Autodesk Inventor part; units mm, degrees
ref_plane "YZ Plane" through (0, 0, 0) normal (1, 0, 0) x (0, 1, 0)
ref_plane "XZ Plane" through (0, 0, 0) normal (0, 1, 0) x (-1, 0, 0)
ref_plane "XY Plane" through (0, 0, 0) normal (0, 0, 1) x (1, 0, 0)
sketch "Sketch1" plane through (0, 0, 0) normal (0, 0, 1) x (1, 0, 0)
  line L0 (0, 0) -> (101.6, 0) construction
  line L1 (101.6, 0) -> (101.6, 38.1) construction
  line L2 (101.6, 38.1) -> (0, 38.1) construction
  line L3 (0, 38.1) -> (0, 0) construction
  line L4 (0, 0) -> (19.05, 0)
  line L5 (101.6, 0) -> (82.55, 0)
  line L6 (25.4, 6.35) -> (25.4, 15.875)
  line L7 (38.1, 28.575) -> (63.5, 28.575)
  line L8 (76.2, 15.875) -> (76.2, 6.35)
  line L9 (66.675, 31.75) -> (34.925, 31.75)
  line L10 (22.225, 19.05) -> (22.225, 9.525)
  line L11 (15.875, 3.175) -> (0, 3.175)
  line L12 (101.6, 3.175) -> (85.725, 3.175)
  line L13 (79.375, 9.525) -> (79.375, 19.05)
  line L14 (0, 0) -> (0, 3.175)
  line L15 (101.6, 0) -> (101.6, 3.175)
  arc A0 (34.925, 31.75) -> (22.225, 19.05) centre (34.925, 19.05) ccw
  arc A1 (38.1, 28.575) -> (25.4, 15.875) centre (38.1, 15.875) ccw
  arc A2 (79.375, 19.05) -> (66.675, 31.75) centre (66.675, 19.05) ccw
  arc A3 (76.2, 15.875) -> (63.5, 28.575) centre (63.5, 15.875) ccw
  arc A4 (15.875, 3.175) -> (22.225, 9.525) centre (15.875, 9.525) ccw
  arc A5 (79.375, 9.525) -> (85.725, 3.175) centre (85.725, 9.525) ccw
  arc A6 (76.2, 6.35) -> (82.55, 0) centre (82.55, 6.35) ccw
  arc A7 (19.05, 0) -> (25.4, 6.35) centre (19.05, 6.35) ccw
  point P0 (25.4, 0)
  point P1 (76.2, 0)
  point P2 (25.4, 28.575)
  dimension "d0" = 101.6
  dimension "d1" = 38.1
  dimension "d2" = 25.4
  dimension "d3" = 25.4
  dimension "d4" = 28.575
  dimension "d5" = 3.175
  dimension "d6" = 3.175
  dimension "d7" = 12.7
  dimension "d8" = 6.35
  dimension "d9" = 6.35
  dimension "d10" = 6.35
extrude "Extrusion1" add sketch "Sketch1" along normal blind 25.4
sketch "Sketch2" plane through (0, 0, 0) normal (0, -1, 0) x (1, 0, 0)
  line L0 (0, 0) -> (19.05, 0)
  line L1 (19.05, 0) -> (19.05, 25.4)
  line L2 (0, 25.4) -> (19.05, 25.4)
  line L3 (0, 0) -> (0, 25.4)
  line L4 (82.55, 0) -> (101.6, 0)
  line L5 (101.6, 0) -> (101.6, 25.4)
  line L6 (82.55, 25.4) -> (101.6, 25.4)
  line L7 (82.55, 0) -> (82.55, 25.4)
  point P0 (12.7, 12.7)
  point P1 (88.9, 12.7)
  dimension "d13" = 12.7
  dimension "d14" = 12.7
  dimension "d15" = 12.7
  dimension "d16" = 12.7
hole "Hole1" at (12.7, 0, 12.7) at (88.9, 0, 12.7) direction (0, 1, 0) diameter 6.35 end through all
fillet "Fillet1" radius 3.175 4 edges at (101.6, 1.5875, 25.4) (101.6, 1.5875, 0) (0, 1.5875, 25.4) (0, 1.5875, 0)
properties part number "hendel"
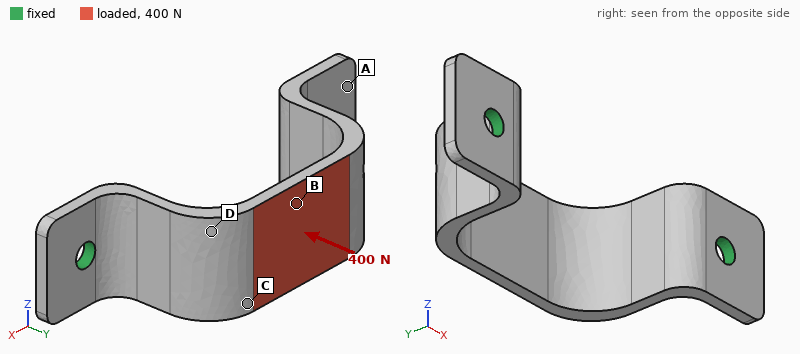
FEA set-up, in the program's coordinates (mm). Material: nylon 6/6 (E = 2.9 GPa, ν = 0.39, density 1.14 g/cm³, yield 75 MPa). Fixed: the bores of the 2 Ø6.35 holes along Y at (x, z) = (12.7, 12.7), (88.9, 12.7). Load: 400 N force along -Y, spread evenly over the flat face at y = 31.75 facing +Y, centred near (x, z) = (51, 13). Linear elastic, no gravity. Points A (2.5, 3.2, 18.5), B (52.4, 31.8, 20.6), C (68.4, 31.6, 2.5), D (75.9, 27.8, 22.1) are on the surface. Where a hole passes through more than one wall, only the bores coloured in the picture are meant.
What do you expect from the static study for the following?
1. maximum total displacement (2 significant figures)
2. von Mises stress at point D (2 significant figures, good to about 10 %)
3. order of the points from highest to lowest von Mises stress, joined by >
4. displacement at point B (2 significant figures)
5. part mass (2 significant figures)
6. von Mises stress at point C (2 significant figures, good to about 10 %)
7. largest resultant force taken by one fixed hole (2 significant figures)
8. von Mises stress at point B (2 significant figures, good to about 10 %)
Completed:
0.90 mm
13 MPa
B > D > C > A
0.84 mm
14 g
9.4 MPa
250 N
25 MPa
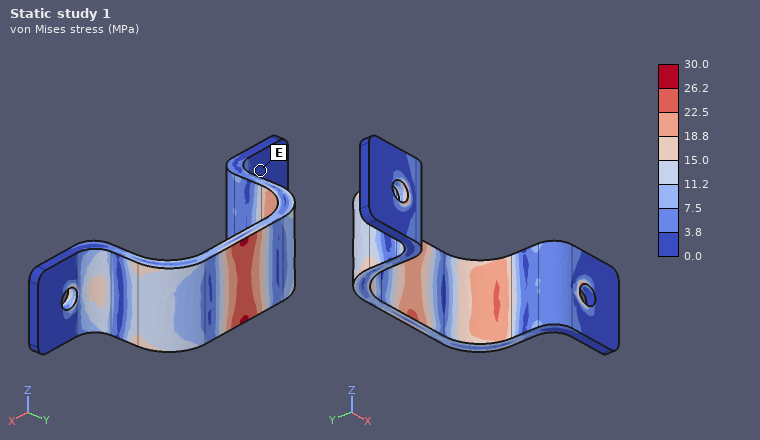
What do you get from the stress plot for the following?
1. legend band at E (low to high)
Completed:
0.0 to 3.8 MPa
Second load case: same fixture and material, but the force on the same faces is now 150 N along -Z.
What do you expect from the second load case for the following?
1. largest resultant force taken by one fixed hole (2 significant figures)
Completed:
75 N
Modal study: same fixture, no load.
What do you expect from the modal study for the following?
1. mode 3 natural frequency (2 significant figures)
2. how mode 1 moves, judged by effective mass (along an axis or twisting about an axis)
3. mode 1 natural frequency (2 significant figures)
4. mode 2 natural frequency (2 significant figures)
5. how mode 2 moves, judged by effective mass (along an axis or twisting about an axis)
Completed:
1200 Hz
along Z
740 Hz
890 Hz
along X
